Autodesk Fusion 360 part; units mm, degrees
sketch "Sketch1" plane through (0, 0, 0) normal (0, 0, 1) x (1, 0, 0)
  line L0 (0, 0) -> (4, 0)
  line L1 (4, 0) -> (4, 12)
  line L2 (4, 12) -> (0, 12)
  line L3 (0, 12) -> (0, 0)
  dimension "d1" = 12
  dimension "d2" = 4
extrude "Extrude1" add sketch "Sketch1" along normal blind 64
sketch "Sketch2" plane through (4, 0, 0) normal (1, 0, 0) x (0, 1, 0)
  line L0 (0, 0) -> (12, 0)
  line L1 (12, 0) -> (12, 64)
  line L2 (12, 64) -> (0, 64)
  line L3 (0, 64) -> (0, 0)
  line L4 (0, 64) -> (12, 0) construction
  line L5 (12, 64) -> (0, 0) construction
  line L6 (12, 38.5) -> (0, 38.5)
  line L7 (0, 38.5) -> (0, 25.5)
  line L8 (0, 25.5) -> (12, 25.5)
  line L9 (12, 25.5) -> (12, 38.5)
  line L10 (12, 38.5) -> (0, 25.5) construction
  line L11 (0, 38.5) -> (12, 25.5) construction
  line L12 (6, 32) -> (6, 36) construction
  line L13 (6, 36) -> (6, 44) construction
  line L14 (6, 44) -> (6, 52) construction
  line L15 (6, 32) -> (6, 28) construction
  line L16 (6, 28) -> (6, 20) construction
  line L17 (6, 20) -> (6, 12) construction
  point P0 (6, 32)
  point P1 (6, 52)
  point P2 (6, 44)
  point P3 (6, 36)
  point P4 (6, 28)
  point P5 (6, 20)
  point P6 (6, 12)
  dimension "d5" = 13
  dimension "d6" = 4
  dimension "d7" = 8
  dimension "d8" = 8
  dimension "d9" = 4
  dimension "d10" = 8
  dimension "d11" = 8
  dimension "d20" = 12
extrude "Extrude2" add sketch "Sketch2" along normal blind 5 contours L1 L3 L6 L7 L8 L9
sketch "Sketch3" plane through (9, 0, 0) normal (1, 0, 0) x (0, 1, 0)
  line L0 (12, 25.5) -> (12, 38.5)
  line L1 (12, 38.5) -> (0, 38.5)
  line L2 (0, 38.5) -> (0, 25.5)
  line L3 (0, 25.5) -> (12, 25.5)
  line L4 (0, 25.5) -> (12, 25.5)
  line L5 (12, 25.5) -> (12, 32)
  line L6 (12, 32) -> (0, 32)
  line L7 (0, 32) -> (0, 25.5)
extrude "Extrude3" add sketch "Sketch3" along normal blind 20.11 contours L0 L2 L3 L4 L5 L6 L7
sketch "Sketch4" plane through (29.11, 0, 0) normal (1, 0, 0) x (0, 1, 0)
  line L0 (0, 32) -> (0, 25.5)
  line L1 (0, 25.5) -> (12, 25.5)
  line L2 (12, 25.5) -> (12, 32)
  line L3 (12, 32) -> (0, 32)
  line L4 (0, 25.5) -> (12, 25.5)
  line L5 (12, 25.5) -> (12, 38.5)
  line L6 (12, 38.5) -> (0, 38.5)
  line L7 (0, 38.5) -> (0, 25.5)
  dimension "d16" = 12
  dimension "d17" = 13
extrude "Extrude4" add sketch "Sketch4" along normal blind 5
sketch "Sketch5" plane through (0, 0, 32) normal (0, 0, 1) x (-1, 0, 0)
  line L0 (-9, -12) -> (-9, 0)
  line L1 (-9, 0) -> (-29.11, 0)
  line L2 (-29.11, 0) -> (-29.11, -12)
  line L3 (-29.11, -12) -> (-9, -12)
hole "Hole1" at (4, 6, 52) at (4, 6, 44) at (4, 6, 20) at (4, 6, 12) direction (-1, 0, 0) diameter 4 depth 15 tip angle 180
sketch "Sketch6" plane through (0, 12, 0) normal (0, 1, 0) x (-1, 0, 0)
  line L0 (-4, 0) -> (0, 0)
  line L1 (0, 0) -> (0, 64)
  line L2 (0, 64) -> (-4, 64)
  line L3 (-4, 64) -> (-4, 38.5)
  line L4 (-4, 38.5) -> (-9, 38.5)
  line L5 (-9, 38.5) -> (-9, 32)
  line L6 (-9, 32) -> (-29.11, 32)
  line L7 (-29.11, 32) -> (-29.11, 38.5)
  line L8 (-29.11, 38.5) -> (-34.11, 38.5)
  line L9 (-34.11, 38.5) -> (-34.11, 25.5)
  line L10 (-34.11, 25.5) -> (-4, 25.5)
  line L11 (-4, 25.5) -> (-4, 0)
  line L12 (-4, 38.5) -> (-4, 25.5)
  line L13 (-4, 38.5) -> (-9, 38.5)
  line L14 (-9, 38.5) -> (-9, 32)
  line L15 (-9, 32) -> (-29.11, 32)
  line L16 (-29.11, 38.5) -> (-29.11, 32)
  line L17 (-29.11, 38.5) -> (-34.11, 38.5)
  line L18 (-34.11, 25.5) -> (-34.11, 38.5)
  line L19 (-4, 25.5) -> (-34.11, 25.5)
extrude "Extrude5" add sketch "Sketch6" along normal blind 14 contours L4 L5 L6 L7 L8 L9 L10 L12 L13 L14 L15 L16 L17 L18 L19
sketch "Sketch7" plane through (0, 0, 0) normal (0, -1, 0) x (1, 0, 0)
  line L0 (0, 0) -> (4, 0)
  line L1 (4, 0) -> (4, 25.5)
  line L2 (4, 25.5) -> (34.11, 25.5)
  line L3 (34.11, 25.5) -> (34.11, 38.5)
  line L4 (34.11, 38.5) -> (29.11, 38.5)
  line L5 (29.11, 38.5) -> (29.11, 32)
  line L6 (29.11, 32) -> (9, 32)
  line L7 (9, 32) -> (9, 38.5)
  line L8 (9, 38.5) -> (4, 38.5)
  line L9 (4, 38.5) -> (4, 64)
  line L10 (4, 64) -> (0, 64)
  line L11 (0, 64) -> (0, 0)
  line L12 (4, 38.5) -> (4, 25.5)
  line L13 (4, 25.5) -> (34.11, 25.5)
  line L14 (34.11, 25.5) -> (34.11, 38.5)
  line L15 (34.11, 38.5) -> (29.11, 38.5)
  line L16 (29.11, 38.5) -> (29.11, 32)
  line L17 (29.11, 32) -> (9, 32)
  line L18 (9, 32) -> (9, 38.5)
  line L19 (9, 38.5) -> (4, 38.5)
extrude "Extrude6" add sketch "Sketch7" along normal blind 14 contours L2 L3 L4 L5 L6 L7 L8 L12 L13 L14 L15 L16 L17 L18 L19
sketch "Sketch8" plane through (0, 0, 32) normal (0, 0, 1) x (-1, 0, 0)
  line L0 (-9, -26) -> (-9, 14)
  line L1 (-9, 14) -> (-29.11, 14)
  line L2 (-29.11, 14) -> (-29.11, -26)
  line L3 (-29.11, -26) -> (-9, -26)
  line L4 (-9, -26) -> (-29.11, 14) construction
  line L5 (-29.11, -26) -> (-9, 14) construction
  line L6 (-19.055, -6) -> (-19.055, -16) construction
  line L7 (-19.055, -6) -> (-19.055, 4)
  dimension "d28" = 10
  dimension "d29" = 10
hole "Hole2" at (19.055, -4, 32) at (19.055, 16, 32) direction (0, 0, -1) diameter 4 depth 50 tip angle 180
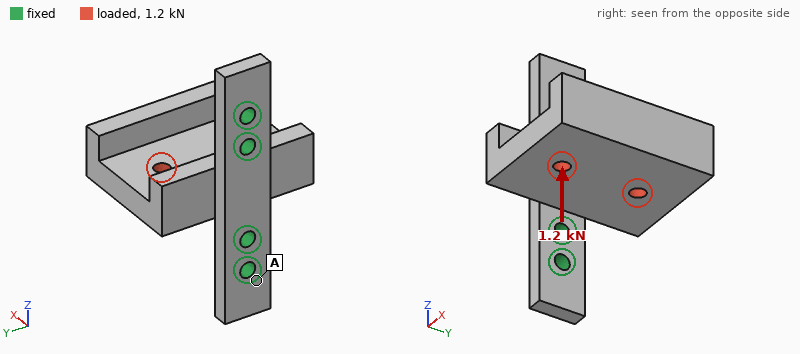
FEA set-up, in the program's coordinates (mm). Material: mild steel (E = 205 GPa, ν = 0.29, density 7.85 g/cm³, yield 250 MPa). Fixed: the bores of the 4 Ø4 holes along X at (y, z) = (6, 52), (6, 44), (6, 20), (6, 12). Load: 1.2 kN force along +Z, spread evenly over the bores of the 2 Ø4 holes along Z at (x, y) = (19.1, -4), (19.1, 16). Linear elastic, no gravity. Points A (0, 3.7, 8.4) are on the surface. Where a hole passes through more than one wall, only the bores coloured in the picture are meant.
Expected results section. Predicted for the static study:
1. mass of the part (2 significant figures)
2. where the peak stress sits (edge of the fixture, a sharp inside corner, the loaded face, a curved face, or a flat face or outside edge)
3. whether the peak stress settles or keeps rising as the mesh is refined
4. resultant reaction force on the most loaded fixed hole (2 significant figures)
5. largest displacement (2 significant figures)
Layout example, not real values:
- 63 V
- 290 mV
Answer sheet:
- 100 g
- edge of the fixture
- keeps rising
- 1.4 kN
- 39 µm
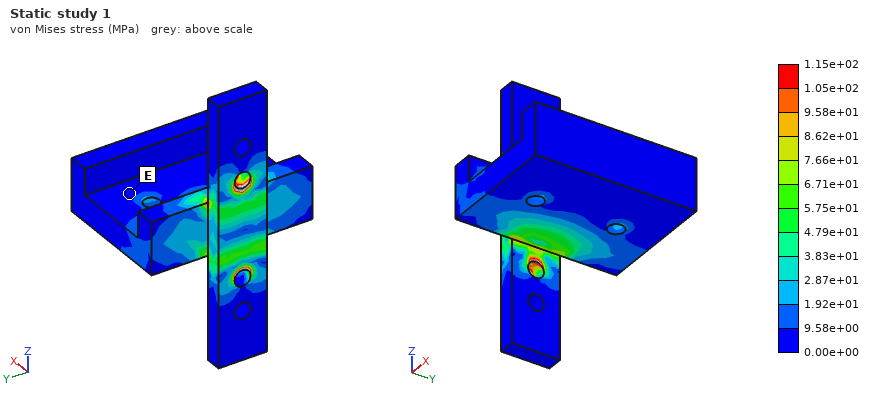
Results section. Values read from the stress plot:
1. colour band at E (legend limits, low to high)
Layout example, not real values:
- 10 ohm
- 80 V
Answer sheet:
- 0.00e+00 to 9.58e+00 MPa
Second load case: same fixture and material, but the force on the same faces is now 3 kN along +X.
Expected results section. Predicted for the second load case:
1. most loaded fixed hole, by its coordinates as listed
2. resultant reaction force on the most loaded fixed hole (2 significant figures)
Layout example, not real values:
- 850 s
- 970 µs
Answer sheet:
- (6, 20)
- 2.2 kN
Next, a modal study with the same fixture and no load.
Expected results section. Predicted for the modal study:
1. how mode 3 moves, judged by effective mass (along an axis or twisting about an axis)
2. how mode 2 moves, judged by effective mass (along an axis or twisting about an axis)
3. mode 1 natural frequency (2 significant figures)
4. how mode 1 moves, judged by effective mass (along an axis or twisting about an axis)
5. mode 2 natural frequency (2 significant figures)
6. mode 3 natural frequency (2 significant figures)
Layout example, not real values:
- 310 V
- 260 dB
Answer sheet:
- twisting about X
- along Z
- 2000 Hz
- along Y
- 3500 Hz
- 6800 Hz
